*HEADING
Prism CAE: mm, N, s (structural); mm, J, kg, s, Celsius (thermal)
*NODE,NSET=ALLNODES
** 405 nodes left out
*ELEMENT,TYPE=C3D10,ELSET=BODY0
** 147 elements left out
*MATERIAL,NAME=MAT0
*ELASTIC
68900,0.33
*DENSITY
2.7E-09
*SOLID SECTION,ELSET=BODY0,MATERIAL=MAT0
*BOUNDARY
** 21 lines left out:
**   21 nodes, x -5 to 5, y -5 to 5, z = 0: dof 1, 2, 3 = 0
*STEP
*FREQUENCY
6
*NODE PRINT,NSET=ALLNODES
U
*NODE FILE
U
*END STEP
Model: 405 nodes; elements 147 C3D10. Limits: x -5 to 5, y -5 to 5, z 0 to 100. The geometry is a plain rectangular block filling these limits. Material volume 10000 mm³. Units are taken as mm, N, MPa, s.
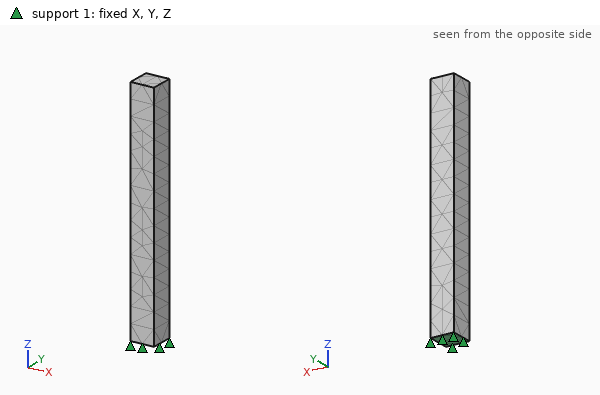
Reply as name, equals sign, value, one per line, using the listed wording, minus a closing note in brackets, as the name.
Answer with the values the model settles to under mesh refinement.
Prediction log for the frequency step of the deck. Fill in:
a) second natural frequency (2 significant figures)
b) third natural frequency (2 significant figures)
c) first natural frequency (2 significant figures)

second natural frequency = 820 Hz
third natural frequency = 4900 Hz
first natural frequency = 820 Hz
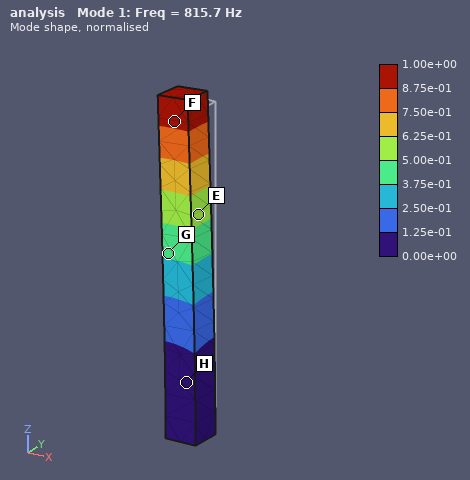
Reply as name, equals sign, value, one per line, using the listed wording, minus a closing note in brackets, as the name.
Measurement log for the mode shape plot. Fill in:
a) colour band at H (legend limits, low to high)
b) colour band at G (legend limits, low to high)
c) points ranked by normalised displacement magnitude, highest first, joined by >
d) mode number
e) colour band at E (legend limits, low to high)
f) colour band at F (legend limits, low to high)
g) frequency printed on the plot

colour band at H = 0.00e+00 to 1.25e-01
colour band at G = 3.75e-01 to 5.00e-01
points ranked by normalised displacement magnitude, highest first, joined by > = F > E > G > H
mode number = 1
colour band at E = 5.00e-01 to 6.25e-01
colour band at F = 8.75e-01 to 1.00e+00
frequency printed on the plot = 815.7 Hz
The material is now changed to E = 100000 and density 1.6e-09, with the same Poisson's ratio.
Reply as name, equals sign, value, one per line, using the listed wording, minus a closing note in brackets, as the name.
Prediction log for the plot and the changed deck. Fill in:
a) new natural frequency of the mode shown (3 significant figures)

new natural frequency of the mode shown = 1280 Hz
